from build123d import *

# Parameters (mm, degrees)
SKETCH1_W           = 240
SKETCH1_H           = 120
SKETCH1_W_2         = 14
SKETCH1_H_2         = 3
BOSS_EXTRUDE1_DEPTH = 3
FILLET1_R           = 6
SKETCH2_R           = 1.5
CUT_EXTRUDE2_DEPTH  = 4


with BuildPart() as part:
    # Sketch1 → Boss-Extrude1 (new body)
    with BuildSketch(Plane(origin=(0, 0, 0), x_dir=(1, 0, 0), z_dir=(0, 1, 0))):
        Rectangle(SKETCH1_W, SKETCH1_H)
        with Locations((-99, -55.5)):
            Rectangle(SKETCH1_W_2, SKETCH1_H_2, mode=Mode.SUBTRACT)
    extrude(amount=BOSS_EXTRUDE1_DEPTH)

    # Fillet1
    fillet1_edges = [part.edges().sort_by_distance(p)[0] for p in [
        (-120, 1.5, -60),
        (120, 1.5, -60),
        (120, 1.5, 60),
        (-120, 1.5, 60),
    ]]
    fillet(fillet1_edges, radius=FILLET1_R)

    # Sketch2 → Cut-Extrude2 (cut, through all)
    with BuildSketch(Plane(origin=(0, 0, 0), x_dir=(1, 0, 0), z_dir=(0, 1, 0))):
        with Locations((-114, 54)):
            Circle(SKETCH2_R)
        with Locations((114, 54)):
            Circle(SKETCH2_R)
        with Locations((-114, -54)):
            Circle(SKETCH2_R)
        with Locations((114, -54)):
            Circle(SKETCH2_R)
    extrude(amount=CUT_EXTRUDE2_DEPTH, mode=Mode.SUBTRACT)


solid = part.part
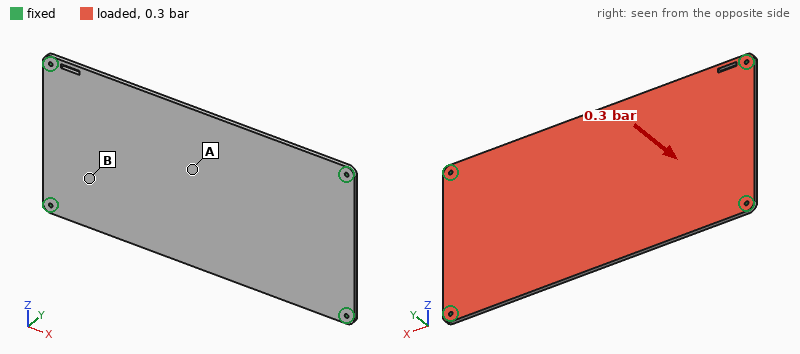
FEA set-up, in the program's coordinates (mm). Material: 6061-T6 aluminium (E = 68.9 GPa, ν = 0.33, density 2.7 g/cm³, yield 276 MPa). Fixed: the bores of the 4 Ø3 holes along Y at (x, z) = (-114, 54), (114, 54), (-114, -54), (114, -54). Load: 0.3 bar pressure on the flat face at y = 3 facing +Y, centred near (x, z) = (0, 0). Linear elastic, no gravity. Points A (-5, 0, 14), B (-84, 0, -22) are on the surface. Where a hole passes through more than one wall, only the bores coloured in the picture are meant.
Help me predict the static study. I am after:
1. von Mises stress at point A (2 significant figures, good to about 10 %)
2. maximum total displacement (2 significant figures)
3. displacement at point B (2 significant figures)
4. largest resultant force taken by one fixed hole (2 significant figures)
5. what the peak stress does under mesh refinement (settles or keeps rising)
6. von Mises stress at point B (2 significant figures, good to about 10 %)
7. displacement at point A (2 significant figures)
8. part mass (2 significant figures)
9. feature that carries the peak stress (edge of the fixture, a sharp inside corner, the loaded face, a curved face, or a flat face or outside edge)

51 MPa
2.3 mm
0.76 mm
220 N
keeps rising
19 MPa
2.2 mm
230 g
edge of the fixture
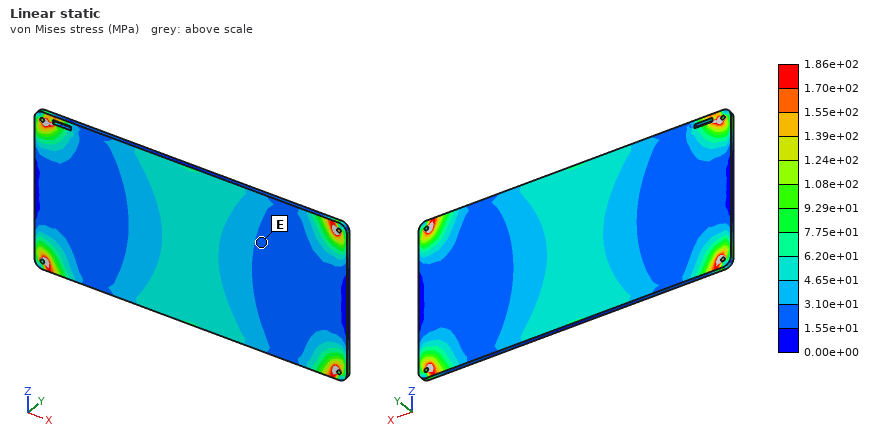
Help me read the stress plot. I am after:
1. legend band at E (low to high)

1.55e+01 to 3.10e+01 MPa
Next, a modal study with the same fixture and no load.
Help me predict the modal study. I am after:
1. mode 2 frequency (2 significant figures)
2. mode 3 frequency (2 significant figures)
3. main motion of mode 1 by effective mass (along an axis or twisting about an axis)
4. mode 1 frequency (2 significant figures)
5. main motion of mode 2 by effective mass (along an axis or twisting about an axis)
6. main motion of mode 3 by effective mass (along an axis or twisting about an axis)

460 Hz
670 Hz
along Y
230 Hz
twisting about X
twisting about Z
